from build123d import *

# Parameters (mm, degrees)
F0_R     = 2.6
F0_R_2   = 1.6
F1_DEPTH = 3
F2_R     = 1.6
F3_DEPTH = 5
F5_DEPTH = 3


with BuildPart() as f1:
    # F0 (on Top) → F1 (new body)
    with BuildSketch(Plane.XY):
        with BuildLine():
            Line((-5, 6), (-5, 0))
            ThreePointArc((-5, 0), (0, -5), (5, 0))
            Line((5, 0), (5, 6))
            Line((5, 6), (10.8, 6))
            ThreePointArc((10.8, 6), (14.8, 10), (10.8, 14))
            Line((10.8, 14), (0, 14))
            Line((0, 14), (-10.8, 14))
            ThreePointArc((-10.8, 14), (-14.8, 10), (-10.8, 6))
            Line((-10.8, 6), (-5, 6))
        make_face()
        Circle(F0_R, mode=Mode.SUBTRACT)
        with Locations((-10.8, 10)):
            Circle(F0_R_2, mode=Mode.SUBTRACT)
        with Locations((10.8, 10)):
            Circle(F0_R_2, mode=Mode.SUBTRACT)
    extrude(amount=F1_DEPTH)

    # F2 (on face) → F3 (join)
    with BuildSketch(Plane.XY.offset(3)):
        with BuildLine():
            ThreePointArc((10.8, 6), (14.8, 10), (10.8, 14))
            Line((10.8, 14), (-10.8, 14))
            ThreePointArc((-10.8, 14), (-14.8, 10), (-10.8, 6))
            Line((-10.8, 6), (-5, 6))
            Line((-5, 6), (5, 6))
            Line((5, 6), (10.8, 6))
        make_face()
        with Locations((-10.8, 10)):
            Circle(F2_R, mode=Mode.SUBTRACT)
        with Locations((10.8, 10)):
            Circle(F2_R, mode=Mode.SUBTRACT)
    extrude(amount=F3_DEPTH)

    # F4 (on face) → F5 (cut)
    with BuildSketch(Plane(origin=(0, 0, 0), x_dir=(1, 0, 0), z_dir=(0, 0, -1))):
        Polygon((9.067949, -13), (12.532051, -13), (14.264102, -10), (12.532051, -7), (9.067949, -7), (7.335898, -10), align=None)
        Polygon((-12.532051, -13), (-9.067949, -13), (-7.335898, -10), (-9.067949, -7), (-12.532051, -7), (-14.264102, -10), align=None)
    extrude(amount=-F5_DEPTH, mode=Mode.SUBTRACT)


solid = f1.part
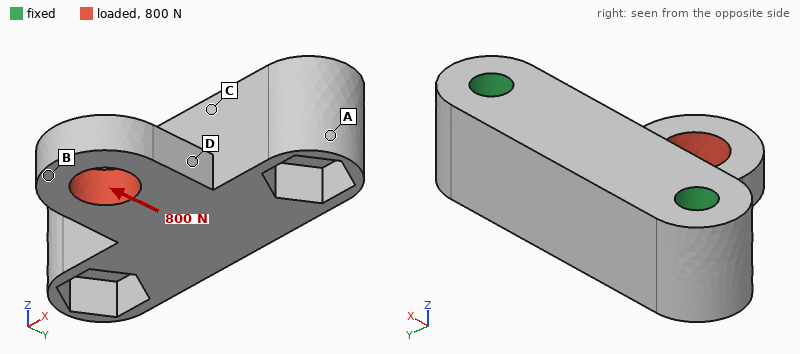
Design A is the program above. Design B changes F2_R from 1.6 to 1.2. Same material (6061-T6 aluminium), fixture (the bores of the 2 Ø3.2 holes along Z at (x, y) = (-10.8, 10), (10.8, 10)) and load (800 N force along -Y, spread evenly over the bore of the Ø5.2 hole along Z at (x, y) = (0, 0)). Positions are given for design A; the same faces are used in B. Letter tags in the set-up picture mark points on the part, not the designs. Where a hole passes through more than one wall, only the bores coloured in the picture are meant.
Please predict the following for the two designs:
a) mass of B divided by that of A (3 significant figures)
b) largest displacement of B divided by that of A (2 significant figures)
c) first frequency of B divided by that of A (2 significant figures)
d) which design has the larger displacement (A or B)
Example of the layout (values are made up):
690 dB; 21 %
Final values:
1.02; 1.1; 0.98; B
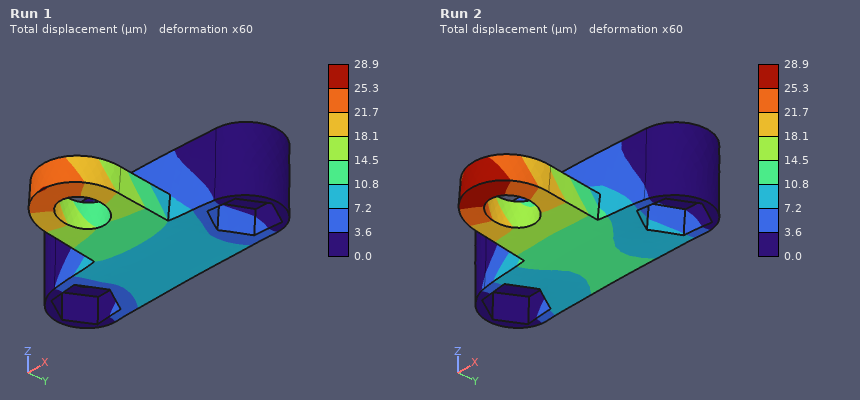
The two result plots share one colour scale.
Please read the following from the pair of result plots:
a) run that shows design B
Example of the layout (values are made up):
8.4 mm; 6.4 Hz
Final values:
Run 2
